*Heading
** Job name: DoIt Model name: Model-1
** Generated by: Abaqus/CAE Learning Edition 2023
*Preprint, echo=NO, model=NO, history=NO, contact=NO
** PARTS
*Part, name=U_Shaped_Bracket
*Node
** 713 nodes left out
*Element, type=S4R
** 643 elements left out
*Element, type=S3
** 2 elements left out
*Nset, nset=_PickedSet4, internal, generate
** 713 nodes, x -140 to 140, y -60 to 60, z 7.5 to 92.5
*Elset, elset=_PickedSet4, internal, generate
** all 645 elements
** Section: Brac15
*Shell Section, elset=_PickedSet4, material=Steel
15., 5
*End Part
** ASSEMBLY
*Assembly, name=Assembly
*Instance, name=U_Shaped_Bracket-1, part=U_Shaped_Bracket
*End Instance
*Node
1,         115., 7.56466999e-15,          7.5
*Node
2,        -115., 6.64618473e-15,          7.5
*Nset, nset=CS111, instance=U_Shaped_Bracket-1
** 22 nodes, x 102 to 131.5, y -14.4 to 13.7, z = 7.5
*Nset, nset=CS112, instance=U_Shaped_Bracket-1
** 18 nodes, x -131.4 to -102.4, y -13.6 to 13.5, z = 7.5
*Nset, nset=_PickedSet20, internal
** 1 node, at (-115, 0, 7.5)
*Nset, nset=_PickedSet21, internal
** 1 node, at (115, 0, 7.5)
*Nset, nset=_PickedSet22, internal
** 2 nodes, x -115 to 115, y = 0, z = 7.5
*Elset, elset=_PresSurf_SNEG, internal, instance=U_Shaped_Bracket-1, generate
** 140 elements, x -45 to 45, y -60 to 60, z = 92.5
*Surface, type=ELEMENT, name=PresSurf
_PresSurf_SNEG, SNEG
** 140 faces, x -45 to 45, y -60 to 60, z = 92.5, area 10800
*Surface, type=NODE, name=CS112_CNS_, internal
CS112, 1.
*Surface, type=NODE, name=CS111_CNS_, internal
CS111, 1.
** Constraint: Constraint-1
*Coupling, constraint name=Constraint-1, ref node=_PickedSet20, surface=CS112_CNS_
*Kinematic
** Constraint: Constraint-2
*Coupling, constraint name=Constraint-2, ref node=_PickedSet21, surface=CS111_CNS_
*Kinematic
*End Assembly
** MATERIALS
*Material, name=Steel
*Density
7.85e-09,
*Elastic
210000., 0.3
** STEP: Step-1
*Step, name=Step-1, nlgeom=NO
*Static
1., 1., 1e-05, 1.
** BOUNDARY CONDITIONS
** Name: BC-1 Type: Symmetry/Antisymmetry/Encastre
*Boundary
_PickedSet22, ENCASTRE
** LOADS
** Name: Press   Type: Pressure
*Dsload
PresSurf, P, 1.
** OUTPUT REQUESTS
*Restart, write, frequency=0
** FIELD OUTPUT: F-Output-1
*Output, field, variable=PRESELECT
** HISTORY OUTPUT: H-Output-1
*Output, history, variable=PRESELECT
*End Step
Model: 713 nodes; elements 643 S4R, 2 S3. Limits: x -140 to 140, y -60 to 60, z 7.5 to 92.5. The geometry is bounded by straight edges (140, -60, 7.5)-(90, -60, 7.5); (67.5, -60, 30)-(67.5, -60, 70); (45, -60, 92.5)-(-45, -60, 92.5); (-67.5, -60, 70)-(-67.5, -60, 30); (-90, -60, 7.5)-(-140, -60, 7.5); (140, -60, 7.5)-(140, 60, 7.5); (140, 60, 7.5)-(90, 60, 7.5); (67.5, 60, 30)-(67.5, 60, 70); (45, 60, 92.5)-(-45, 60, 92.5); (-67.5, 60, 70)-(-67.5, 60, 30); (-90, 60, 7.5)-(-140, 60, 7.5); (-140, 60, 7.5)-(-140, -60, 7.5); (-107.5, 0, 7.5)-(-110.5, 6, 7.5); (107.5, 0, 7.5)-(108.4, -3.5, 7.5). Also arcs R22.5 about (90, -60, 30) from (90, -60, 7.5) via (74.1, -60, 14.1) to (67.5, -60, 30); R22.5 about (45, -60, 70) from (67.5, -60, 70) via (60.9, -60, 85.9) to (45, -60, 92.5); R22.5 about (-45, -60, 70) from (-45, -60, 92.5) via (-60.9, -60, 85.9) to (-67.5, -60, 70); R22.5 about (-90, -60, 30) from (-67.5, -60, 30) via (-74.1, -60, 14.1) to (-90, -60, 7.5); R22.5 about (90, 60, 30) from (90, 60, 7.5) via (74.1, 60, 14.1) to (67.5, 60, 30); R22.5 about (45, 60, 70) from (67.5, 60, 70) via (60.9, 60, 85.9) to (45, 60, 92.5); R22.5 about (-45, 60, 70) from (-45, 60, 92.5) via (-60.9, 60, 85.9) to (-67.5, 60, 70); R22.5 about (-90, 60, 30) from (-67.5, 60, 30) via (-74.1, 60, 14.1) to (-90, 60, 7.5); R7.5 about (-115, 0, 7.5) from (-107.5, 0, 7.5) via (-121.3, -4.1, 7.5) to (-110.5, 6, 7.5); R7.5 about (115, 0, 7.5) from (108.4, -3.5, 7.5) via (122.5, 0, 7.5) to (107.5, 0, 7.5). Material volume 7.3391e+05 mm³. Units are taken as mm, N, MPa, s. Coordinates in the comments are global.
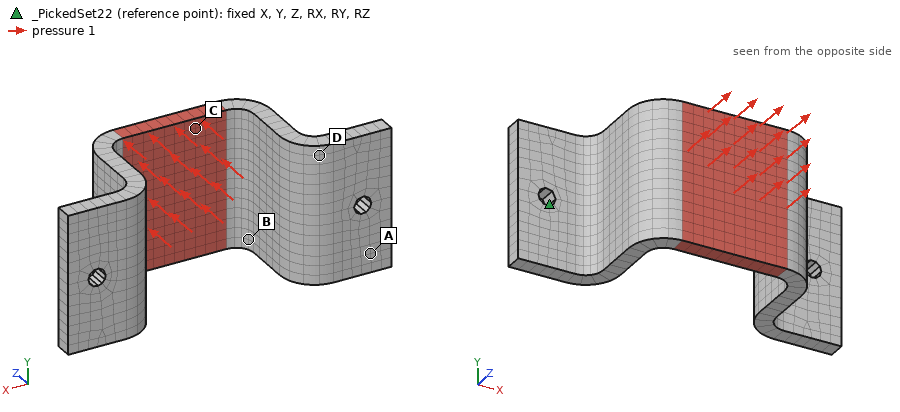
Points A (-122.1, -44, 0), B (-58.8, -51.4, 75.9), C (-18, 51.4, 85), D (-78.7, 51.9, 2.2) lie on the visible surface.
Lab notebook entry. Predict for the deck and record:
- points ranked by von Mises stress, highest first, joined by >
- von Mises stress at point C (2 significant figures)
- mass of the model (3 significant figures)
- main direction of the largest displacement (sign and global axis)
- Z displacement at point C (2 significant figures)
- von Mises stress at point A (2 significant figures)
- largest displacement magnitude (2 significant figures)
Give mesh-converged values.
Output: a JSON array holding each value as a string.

["B > C > D > A", "15 MPa", "5.76 kg", "+Z", "0.029 mm", "4.4 MPa", "0.032 mm"]
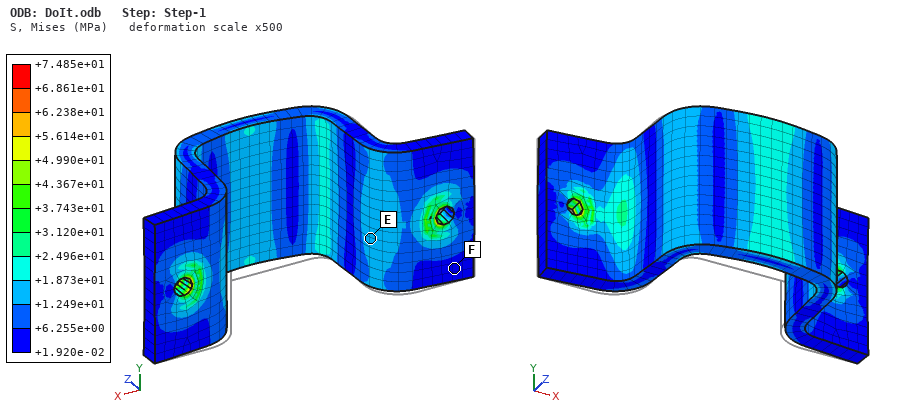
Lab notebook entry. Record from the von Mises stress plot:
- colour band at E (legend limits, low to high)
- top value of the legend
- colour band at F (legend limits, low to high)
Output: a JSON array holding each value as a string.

["+1.249e+01 to +1.873e+01 MPa", "+7.485e+01 MPa", "+1.920e-02 to +6.255e+00 MPa"]
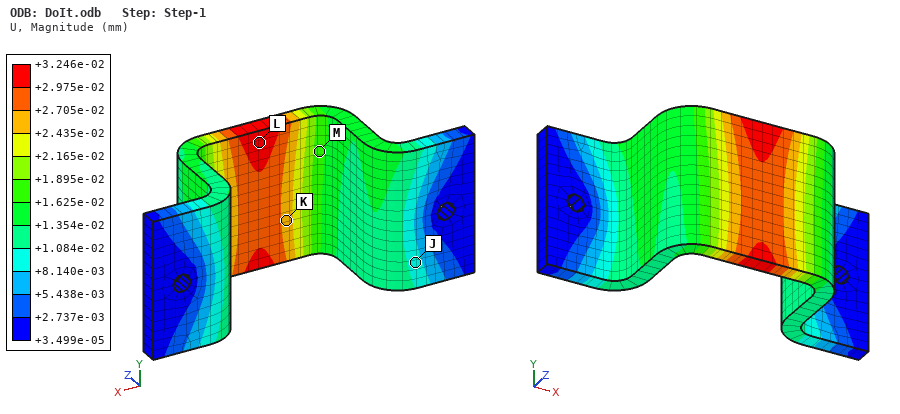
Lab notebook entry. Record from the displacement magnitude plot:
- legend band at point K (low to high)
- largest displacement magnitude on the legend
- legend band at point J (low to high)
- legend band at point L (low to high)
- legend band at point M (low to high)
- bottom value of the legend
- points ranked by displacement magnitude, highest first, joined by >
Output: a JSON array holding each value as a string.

["+2.435e-02 to +2.705e-02 mm", "+3.246e-02 mm", "+8.140e-03 to +1.084e-02 mm", "+2.975e-02 to +3.246e-02 mm", "+1.625e-02 to +1.895e-02 mm", "+3.499e-05 mm", "L > K > M > J"]
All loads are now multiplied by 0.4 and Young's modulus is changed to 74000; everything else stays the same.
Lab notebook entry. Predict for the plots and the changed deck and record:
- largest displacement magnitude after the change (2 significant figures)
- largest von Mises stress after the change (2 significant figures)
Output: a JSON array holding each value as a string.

["0.037 mm", "30 MPa"]
